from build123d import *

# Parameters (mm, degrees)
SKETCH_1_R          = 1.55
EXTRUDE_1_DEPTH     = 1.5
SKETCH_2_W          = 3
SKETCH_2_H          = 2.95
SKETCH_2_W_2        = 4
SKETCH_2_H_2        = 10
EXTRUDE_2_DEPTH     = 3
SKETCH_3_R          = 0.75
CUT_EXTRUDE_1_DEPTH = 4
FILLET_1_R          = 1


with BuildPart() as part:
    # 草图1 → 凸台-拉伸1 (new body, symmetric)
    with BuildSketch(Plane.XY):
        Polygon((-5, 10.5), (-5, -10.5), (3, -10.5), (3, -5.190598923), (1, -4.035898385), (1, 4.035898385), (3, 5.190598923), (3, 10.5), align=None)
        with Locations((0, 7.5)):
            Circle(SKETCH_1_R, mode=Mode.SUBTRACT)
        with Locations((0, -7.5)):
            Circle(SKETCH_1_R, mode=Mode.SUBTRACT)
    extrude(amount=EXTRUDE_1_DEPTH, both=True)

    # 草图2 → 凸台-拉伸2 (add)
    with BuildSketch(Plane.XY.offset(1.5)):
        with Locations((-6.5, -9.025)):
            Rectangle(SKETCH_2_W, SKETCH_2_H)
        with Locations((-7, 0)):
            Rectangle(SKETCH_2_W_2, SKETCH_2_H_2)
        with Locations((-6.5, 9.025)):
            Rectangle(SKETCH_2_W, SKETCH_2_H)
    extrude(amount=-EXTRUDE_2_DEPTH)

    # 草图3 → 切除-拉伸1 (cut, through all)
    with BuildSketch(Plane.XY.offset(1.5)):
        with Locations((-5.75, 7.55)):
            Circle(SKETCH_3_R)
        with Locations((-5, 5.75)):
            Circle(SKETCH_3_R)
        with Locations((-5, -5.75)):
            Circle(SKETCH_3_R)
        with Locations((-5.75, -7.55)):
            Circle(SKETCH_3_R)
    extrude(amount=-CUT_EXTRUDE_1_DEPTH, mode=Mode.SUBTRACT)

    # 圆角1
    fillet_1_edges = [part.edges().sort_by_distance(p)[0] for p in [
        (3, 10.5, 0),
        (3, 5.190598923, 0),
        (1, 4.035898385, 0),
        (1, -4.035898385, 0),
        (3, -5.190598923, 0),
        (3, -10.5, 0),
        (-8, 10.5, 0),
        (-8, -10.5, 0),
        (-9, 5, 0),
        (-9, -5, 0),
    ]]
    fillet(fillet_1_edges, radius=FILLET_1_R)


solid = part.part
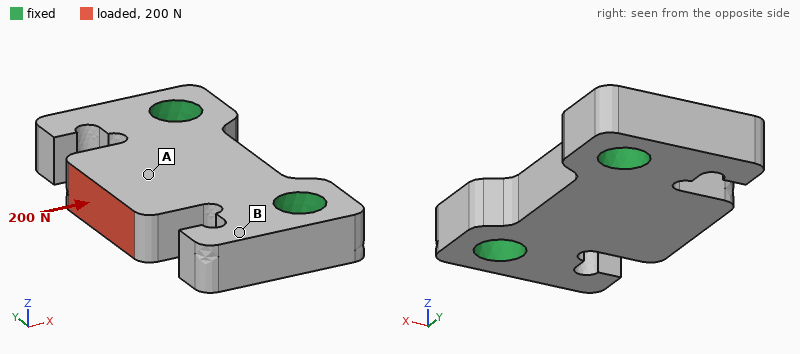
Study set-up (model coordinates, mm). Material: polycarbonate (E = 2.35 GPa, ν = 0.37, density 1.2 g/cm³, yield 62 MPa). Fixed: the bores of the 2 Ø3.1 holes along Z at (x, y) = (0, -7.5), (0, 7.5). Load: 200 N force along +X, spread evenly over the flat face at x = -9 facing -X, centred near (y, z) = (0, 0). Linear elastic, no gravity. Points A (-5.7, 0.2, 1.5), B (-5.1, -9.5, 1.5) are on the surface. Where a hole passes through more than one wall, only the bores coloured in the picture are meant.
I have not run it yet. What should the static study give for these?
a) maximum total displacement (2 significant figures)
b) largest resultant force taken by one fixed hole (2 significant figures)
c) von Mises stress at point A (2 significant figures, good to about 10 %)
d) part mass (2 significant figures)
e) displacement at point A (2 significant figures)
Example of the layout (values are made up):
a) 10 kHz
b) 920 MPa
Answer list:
a) 43 µm
b) 120 N
c) 5.4 MPa
d) 0.67 g
e) 34 µm
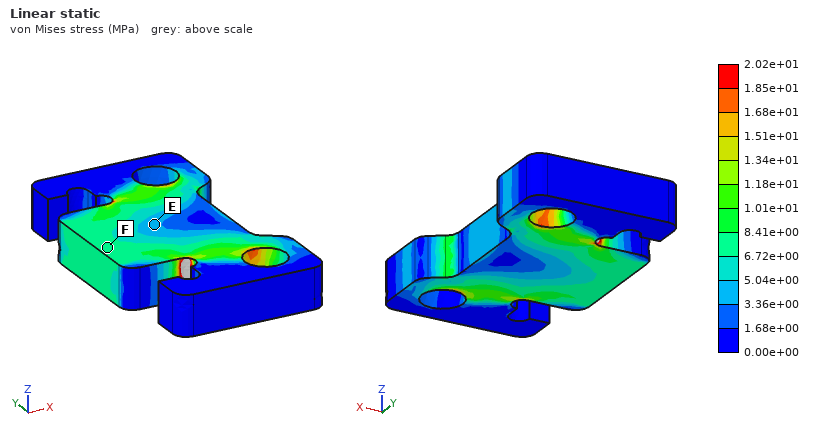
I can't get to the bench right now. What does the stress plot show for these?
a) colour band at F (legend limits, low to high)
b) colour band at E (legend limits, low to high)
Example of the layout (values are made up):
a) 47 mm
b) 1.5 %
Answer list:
a) 6.72e+00 to 8.41e+00 MPa
b) 3.36e+00 to 5.04e+00 MPa
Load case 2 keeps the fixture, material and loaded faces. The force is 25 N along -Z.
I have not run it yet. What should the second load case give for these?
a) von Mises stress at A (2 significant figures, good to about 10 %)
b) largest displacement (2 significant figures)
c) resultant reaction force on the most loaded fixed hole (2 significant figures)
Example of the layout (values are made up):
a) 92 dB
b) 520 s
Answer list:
a) 5.9 MPa
b) 0.14 mm
c) 13 N
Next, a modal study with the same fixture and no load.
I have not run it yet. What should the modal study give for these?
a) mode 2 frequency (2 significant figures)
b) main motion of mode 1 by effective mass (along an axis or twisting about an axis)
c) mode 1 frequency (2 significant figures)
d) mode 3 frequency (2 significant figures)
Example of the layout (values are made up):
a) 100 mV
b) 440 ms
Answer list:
a) 15 kHz
b) along Z
c) 7400 Hz
d) 15 kHz
